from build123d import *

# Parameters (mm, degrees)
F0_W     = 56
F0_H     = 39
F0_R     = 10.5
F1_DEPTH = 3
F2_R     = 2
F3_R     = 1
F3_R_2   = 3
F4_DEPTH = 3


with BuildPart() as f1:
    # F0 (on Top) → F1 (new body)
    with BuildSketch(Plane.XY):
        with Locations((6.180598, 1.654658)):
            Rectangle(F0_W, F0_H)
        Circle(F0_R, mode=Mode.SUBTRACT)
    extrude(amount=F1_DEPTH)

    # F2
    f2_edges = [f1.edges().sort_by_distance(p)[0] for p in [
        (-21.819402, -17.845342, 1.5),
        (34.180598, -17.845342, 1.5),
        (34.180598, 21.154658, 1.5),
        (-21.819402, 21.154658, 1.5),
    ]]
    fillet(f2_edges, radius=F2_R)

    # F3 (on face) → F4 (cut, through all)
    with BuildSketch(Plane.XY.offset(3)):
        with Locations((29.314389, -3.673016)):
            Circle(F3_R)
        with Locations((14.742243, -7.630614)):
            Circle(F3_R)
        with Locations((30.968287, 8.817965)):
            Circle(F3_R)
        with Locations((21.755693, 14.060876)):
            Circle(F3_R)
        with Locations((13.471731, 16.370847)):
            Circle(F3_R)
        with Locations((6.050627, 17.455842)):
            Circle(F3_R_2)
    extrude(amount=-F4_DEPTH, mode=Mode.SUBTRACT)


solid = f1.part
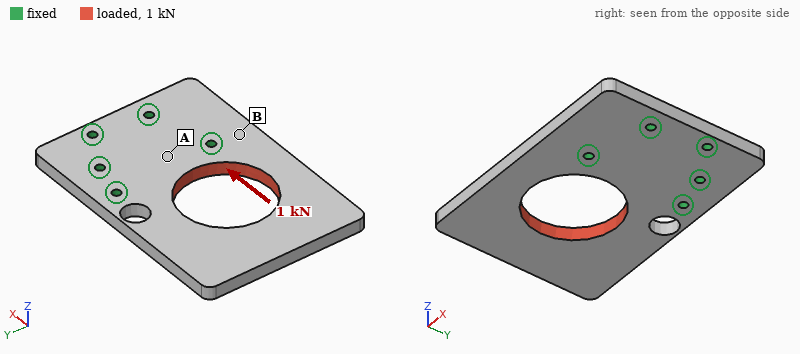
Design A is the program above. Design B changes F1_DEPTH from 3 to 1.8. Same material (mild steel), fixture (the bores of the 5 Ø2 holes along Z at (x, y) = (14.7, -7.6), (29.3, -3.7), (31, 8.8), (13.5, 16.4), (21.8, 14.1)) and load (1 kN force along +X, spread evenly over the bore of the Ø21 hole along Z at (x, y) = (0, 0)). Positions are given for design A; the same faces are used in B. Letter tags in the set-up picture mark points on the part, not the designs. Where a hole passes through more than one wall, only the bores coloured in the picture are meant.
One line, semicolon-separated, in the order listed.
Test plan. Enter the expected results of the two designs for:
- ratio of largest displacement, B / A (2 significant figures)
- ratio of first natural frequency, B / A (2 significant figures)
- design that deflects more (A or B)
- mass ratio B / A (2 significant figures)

1.7; 0.61; B; 0.60
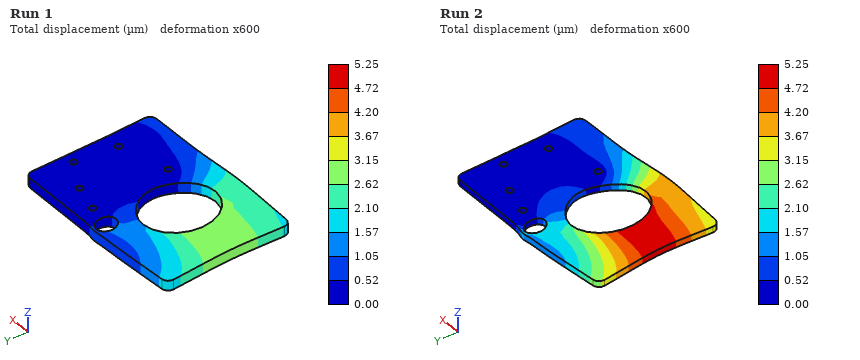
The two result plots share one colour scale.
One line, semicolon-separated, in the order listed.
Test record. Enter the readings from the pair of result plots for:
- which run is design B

Run 2
